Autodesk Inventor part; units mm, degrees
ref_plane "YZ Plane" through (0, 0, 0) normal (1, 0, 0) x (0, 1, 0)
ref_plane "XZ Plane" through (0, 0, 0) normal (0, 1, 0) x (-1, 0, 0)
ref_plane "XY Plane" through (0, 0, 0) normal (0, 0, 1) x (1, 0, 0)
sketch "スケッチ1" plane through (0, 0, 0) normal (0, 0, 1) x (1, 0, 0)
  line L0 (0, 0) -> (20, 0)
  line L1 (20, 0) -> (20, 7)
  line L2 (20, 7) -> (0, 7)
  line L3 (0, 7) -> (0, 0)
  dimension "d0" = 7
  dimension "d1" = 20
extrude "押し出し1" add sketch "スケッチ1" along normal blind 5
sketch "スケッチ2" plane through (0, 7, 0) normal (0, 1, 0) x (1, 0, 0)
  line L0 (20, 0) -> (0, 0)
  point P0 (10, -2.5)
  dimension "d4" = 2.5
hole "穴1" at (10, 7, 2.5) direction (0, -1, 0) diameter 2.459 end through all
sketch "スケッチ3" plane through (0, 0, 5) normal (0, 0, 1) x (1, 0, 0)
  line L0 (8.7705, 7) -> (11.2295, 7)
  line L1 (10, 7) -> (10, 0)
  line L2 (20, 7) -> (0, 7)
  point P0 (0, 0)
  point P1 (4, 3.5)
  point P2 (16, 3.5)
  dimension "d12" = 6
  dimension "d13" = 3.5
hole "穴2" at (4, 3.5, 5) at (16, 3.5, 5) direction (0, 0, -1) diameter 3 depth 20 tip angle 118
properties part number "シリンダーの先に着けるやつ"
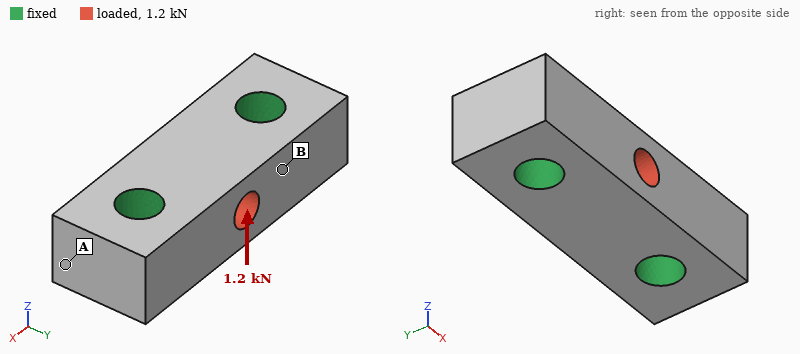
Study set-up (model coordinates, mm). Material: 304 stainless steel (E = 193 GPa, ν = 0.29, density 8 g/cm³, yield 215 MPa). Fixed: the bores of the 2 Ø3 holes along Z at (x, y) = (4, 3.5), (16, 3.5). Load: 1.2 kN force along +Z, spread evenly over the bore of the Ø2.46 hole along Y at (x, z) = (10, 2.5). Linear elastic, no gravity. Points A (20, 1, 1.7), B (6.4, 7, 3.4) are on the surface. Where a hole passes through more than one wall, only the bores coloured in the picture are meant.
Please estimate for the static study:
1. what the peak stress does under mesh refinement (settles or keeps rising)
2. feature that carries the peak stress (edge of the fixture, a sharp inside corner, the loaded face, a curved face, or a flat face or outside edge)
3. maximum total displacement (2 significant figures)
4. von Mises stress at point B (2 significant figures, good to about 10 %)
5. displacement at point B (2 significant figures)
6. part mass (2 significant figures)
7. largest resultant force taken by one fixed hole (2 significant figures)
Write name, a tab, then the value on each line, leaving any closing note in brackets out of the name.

what the peak stress does under mesh refinement	keeps rising
feature that carries the peak stress	edge of the fixture
maximum total displacement	1.9 µm
von Mises stress at point B	29 MPa
displacement at point B	0.65 µm
part mass	4.8 g
largest resultant force taken by one fixed hole	600 N
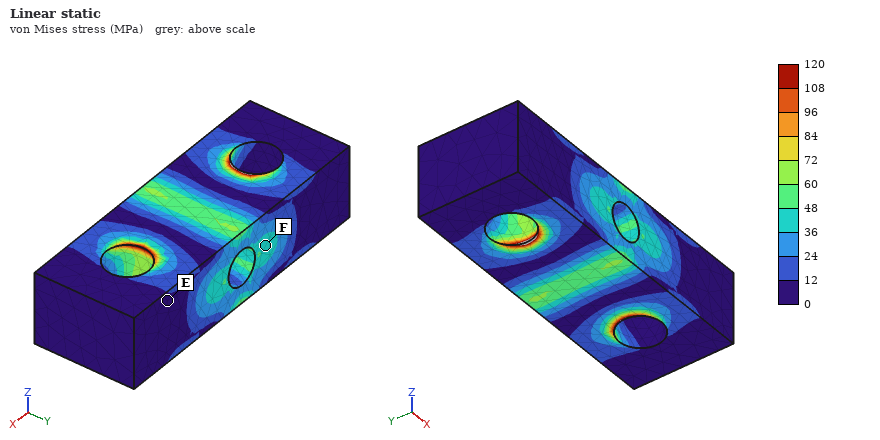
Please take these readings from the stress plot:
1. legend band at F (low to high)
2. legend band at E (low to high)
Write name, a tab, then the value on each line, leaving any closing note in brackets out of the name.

legend band at F	36 to 48 MPa
legend band at E	0 to 12 MPa
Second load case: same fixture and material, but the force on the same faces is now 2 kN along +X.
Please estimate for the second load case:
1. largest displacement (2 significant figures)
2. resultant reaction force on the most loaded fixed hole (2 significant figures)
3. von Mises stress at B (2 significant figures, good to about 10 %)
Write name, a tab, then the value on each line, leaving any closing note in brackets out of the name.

largest displacement	0.89 µm
resultant reaction force on the most loaded fixed hole	1.0 kN
von Mises stress at B	20 MPa
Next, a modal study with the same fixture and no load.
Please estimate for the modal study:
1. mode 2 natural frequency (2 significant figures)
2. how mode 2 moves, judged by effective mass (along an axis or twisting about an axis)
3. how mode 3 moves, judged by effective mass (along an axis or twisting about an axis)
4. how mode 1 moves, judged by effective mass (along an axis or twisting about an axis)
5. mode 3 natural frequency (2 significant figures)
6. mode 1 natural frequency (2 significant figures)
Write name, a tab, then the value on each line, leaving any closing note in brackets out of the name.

mode 2 natural frequency	130 kHz
how mode 2 moves, judged by effective mass	along Z
how mode 3 moves, judged by effective mass	twisting about X
how mode 1 moves, judged by effective mass	along Y
mode 3 natural frequency	130 kHz
mode 1 natural frequency	120 kHz
